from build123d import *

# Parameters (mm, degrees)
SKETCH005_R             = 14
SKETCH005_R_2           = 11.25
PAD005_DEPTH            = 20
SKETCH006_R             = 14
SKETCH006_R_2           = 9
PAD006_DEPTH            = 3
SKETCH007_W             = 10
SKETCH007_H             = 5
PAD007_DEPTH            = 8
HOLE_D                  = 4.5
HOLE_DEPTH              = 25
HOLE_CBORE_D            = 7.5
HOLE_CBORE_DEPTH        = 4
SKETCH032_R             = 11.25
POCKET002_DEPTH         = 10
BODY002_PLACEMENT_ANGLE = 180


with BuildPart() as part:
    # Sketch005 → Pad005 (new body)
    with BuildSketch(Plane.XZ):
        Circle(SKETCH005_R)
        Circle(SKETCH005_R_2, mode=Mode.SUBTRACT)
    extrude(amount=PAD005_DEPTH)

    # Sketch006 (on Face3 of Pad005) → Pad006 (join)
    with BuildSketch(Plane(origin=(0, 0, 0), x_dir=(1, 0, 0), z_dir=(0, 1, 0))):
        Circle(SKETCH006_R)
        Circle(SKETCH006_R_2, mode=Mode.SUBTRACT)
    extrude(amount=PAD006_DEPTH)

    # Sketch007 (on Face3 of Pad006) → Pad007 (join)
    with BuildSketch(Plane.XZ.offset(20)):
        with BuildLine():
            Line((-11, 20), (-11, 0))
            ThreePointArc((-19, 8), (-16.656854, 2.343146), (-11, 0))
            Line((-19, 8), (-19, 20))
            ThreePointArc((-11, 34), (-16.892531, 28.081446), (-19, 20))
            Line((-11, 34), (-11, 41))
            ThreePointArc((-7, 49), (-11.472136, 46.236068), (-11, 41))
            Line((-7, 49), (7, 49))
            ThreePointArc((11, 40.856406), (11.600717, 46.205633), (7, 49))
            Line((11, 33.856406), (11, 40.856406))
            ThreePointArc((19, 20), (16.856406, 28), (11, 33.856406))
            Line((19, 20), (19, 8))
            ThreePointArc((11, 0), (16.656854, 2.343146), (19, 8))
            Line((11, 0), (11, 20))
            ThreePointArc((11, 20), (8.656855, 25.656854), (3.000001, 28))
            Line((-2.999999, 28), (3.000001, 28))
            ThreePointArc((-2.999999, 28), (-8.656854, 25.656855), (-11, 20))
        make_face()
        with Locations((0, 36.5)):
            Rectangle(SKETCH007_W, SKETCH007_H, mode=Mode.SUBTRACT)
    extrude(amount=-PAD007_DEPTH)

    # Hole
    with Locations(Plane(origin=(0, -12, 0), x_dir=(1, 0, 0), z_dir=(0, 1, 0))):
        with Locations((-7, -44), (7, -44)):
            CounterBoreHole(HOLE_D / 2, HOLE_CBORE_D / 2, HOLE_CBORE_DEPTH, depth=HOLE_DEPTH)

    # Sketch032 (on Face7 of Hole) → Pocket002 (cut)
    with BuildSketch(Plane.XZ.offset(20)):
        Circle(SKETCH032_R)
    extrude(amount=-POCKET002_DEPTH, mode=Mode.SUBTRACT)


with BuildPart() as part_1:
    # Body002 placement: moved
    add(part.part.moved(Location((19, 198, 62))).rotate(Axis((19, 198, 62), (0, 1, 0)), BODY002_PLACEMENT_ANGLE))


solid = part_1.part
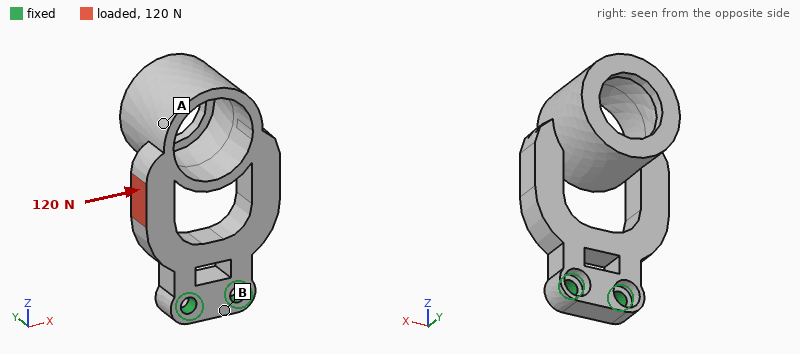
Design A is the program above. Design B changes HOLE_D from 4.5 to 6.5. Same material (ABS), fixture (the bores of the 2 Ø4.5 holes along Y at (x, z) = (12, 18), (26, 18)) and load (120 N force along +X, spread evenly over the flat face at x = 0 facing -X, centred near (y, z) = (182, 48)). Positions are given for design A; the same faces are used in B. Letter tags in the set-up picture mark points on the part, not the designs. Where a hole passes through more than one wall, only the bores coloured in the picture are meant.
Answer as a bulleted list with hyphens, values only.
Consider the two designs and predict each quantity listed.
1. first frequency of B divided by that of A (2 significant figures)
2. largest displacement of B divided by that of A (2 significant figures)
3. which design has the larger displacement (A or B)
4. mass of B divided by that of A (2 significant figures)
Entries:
- 1.1
- 0.92
- A
- 0.99
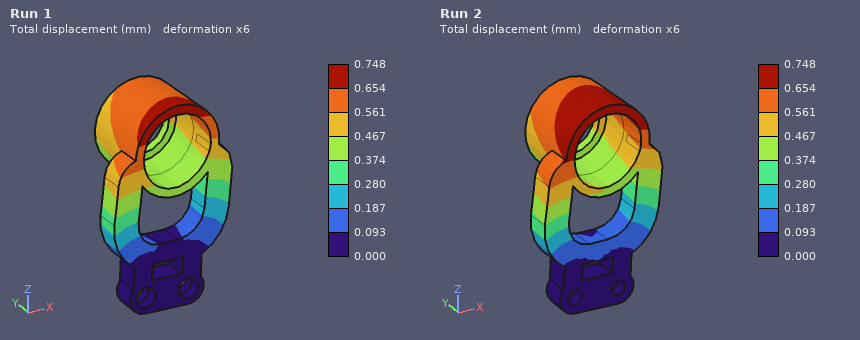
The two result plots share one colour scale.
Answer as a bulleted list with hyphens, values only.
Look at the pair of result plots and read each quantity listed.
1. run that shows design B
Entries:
- Run 1
